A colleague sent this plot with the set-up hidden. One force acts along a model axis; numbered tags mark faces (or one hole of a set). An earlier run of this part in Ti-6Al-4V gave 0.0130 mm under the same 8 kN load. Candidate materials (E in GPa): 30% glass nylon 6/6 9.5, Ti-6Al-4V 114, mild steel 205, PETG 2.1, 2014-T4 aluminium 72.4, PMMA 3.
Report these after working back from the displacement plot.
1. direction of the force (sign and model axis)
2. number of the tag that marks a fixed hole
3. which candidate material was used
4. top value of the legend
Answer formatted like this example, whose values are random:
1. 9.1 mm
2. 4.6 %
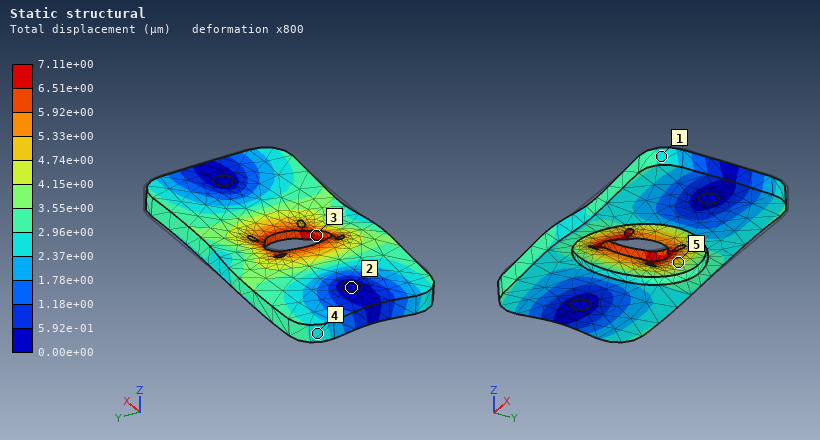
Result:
1. -X
2. 2
3. mild steel
4. 7.11e+00 µm
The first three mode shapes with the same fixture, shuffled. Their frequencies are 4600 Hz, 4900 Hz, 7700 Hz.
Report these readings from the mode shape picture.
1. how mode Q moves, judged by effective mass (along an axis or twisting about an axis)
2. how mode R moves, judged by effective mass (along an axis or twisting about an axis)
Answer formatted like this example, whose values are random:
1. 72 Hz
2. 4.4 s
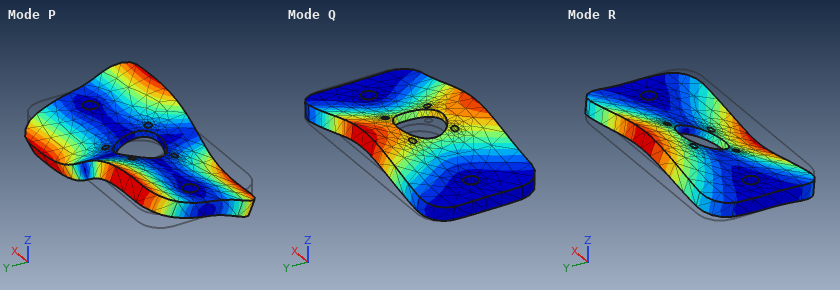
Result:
1. along Z
2. twisting about X
